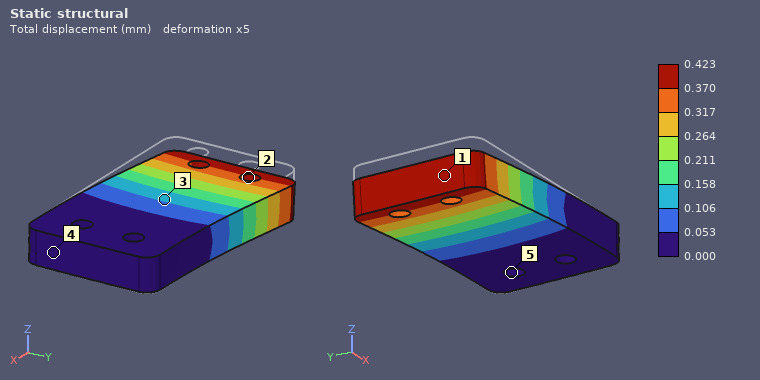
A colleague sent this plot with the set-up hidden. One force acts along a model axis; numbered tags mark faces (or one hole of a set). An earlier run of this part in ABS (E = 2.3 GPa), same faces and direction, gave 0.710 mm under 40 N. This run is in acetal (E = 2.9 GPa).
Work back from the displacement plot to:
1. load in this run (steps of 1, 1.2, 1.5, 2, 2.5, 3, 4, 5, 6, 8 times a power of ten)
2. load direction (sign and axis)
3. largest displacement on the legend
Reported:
30 N
-Z
0.423 mm
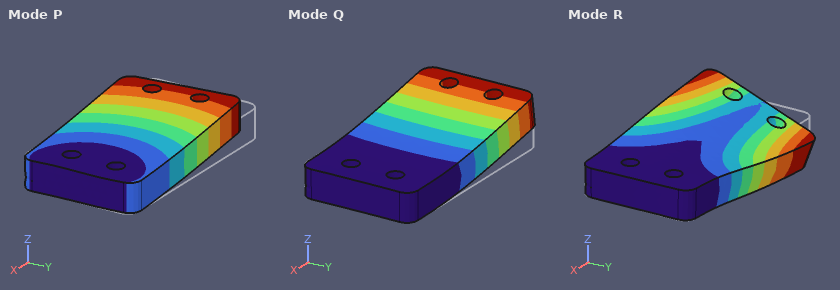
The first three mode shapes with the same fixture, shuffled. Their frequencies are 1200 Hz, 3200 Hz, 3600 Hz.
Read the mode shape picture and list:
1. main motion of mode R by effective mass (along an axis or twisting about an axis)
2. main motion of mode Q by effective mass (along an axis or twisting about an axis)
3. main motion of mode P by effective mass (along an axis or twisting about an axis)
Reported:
twisting about X
along Z
along Y
